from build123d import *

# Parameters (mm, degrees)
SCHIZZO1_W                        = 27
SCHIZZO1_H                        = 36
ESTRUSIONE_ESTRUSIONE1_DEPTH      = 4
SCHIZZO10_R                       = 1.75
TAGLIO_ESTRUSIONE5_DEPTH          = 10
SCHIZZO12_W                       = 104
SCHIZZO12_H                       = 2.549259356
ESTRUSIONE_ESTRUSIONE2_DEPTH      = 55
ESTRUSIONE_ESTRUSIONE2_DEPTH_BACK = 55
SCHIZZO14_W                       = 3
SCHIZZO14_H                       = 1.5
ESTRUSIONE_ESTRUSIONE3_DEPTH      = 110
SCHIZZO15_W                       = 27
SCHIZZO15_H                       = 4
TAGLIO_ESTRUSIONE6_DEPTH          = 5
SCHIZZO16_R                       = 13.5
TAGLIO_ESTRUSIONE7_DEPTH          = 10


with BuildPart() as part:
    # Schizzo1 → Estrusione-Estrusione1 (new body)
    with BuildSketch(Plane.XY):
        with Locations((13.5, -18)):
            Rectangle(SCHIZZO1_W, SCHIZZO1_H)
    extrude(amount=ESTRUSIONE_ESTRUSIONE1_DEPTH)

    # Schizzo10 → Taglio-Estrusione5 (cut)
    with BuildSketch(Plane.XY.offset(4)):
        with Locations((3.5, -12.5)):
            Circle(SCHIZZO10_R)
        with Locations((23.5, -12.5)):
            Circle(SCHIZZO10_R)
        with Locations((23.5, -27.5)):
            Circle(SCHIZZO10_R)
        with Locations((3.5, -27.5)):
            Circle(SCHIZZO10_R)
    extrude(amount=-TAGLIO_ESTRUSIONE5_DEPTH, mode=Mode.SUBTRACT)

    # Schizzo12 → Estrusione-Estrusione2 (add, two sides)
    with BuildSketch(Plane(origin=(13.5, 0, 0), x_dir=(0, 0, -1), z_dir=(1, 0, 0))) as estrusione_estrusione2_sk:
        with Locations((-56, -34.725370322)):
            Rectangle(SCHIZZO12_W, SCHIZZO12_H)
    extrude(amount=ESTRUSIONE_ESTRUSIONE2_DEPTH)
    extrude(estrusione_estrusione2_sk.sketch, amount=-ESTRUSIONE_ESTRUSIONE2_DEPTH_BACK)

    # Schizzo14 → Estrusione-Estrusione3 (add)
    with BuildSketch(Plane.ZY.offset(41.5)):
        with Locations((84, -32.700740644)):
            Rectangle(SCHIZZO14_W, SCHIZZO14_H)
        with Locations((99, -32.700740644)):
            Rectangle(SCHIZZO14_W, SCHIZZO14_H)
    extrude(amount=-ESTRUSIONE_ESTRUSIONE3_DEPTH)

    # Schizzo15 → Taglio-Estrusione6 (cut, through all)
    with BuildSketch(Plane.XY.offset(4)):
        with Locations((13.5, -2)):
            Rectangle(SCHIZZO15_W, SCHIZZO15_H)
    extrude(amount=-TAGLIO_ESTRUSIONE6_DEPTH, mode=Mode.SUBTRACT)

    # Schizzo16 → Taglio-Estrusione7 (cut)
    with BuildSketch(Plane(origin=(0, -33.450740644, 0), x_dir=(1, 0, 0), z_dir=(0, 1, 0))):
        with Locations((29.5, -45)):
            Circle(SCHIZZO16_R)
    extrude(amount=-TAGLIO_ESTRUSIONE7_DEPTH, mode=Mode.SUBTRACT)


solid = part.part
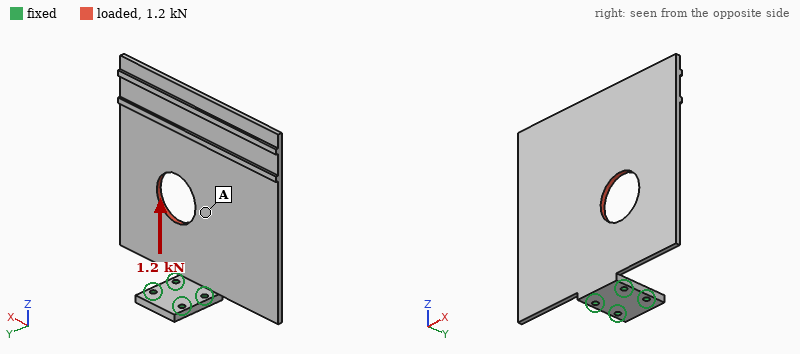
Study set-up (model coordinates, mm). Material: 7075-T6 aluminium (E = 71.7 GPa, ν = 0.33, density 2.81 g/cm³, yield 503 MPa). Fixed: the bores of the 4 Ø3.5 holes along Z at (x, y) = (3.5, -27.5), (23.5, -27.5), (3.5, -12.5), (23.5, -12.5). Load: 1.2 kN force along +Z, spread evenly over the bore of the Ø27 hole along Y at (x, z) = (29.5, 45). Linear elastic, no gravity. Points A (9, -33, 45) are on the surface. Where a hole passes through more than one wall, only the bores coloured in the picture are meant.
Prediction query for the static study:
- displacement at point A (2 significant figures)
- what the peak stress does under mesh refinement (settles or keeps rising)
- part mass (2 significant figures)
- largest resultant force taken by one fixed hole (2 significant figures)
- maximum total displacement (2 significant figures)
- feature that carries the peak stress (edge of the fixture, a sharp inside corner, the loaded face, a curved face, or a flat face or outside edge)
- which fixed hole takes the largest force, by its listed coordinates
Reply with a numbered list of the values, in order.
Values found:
1. 0.17 mm
2. keeps rising
3. 90 g
4. 1.6 kN
5. 0.59 mm
6. edge of the fixture
7. (23.5, -27.5)
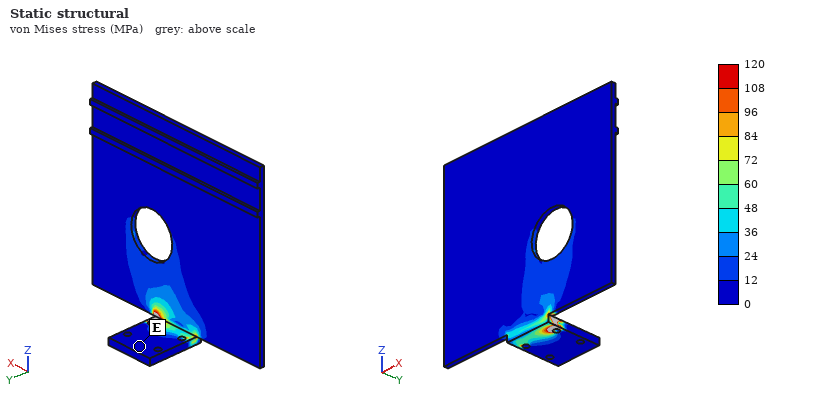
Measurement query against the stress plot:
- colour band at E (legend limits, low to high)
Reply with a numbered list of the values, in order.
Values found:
1. 0 to 12 MPa
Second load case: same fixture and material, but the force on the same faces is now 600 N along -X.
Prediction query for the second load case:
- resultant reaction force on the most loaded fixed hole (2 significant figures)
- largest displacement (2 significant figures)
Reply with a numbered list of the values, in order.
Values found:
1. 1.3 kN
2. 0.50 mm
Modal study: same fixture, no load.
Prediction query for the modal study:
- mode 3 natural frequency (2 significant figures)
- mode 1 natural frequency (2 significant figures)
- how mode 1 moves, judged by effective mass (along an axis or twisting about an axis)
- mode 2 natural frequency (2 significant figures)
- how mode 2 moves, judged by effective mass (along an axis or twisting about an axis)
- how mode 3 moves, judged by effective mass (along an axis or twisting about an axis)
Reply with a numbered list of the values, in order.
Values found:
1. 650 Hz
2. 120 Hz
3. along Y
4. 260 Hz
5. twisting about Z
6. along X
